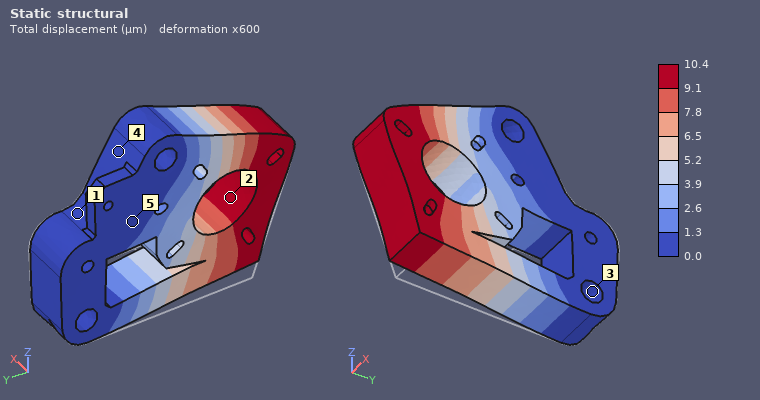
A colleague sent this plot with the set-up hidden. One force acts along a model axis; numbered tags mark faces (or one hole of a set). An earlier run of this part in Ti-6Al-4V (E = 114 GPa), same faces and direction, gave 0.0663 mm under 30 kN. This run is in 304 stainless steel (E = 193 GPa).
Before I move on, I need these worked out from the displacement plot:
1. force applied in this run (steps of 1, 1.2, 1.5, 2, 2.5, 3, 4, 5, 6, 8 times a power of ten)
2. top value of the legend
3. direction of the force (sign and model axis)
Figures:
8 kN
10.4 µm
+Z
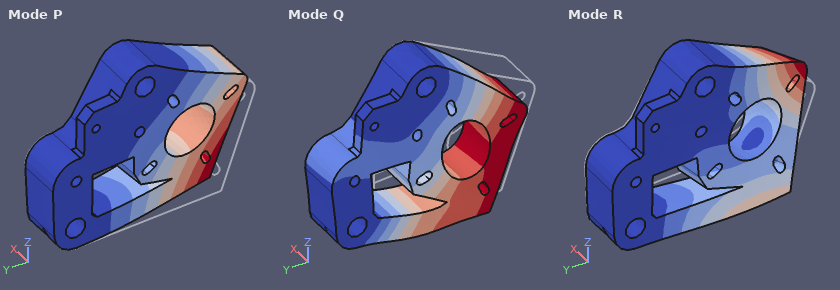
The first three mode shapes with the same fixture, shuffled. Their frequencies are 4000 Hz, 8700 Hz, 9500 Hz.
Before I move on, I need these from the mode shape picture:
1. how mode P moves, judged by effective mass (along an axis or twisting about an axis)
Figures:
along X
